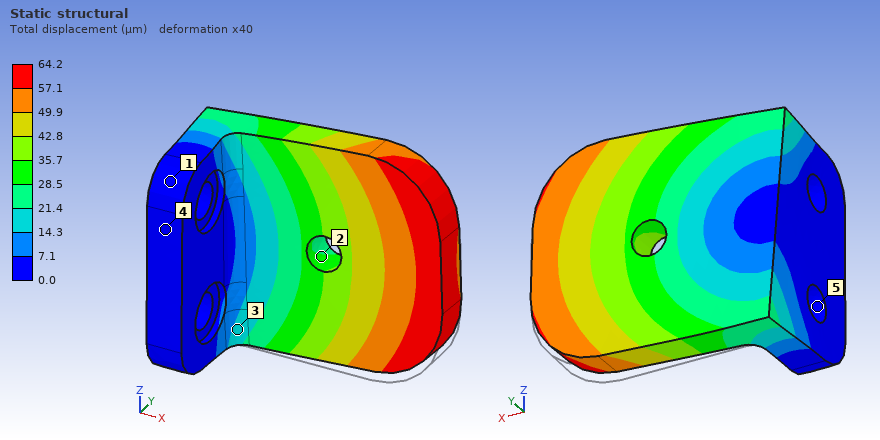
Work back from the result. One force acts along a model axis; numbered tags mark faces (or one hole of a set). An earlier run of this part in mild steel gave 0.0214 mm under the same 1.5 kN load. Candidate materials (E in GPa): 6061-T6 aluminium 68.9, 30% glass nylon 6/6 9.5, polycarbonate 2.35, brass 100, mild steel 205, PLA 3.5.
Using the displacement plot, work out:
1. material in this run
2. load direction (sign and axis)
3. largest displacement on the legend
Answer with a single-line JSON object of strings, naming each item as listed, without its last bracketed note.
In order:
{"material in this run": "6061-T6 aluminium", "load direction": "+Z", "largest displacement on the legend": "64.2 µm"}
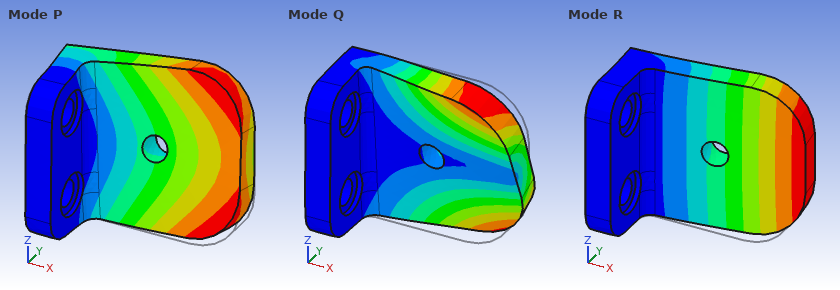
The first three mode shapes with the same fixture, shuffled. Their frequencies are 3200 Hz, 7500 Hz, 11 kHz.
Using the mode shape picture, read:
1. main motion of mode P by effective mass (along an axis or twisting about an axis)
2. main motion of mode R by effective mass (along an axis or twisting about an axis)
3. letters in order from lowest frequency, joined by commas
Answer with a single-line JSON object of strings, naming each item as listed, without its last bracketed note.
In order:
{"main motion of mode P by effective mass": "along Z", "main motion of mode R by effective mass": "along Y", "letters in order from lowest frequency, joined by commas": "R, P, Q"}
